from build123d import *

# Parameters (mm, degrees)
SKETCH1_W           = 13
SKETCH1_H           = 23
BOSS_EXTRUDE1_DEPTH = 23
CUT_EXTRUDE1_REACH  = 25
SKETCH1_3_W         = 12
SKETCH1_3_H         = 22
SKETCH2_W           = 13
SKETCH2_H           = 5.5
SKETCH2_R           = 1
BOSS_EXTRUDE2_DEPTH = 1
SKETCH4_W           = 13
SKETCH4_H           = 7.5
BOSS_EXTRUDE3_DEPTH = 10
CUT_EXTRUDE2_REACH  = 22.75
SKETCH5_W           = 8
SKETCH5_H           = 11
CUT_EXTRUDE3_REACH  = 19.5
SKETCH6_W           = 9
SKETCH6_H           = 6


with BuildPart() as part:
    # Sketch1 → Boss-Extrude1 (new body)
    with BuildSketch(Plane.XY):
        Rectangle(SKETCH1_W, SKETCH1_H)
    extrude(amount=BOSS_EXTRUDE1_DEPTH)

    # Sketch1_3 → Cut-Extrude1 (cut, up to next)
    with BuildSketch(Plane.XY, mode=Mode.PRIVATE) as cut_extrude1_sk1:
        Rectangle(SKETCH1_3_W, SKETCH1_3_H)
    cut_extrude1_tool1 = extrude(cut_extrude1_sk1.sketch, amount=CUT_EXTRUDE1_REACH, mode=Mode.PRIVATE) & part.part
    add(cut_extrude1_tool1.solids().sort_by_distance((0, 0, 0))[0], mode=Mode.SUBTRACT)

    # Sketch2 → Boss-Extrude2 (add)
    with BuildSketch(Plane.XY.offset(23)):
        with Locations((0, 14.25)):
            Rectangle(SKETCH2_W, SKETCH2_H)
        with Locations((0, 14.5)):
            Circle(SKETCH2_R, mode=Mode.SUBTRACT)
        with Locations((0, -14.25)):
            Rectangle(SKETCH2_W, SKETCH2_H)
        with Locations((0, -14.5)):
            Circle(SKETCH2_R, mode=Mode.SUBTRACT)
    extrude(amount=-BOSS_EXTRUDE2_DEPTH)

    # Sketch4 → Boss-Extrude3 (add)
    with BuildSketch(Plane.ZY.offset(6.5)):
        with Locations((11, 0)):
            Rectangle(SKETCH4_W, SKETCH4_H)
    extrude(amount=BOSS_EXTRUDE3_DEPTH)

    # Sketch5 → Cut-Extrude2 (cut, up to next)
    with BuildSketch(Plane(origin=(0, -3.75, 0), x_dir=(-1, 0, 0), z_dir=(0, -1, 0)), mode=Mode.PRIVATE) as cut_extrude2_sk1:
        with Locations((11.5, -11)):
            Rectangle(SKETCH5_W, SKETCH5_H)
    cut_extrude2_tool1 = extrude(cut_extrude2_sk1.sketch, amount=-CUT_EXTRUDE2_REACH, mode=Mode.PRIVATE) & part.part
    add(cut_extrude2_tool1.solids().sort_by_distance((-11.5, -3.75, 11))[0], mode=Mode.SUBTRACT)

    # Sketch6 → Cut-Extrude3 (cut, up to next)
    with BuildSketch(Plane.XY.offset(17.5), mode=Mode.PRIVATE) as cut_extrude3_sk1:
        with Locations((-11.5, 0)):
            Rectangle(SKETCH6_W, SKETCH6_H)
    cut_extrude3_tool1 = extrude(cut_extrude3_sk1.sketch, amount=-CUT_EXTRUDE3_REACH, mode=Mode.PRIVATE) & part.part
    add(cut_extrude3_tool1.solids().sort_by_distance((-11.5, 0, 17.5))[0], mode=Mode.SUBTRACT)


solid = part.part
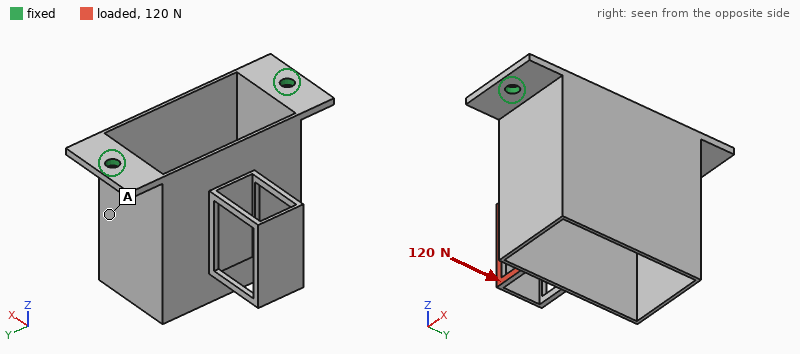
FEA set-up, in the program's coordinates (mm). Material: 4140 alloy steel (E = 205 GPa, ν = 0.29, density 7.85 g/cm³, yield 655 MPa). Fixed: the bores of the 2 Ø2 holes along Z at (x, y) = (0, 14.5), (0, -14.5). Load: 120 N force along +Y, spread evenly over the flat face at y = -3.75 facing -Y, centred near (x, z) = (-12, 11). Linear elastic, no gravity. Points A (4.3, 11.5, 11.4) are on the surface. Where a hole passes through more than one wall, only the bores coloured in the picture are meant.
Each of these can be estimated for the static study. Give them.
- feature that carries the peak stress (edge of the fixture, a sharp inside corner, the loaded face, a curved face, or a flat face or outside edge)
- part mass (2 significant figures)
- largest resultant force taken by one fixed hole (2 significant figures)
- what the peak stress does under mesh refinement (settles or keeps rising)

a sharp inside corner
8.5 g
90 N
keeps rising
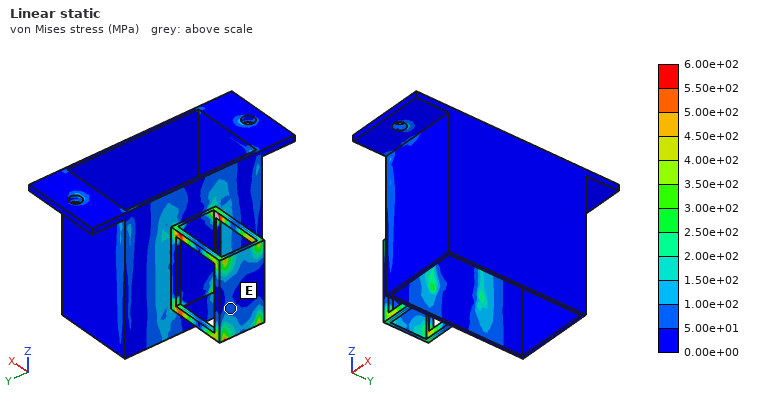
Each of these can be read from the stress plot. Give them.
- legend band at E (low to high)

5.00e+01 to 1.00e+02 MPa
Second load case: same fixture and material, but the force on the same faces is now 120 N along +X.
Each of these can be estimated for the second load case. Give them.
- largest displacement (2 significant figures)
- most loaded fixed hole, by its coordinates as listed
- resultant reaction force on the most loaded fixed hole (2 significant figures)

0.29 mm
(0, -14.5)
84 N
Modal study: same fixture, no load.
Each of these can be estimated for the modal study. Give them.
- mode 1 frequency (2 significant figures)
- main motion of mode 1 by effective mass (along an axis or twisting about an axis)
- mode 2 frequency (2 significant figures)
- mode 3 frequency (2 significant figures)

1800 Hz
along X
3200 Hz
3400 Hz
